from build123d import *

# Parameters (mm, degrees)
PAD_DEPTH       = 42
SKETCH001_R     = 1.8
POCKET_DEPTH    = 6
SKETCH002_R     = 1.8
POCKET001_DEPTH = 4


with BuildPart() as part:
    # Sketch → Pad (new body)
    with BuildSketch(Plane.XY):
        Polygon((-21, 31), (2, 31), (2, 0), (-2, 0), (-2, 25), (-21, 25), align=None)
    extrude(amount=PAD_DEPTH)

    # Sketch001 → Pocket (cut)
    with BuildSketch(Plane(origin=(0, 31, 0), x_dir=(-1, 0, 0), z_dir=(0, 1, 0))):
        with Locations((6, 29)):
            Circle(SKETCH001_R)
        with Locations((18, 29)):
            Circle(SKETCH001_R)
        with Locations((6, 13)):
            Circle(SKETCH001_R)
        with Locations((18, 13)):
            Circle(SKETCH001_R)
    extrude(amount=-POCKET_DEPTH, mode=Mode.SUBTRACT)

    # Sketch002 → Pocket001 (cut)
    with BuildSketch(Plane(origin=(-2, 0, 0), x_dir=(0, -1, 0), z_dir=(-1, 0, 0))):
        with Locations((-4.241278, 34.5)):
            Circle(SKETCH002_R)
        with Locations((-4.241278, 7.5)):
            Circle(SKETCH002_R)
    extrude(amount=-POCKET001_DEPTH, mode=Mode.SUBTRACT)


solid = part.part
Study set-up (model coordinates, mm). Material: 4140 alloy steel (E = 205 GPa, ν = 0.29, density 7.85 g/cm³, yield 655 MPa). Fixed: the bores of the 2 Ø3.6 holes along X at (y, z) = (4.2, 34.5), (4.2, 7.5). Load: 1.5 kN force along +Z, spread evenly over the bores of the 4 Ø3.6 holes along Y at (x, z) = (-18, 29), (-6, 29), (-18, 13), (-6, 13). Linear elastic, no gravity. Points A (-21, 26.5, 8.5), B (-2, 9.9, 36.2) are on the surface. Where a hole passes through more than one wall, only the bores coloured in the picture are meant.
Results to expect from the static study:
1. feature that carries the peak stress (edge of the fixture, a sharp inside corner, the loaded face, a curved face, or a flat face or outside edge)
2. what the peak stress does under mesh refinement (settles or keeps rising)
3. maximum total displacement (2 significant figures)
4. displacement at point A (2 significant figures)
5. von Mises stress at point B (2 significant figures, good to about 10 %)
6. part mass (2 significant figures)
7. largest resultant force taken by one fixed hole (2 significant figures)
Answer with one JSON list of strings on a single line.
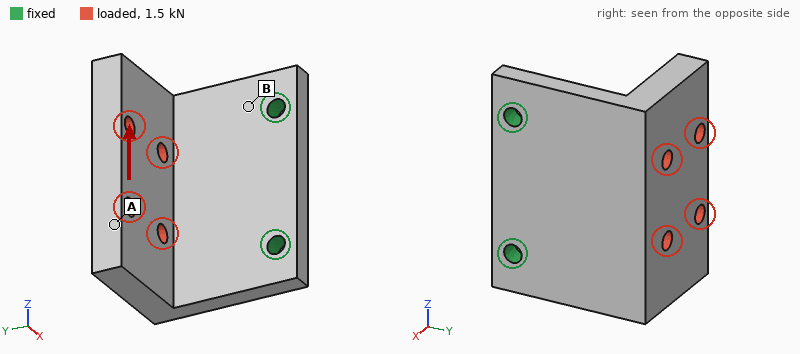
["edge of the fixture", "keeps rising", "74 µm", "62 µm", "77 MPa", "76 g", "1.5 kN"]
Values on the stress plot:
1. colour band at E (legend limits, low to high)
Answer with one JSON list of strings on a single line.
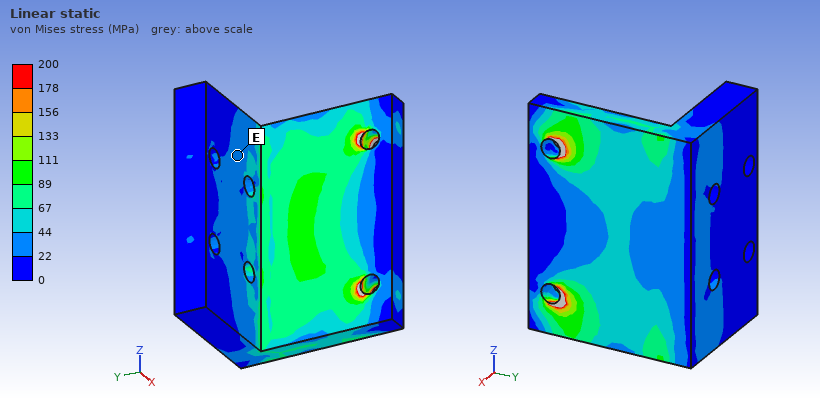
["22 to 44 MPa"]
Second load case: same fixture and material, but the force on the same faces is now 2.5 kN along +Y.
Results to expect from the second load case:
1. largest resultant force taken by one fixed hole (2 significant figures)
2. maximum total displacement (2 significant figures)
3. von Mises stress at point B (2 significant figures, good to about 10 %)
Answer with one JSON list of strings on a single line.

["1.3 kN", "0.42 mm", "320 MPa"]
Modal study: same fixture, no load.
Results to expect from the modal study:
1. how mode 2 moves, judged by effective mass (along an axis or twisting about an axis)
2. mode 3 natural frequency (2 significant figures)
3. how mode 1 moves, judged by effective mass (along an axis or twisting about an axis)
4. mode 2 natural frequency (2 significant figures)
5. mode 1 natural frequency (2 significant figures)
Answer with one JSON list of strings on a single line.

["along Z", "6400 Hz", "along X", "3700 Hz", "1800 Hz"]
